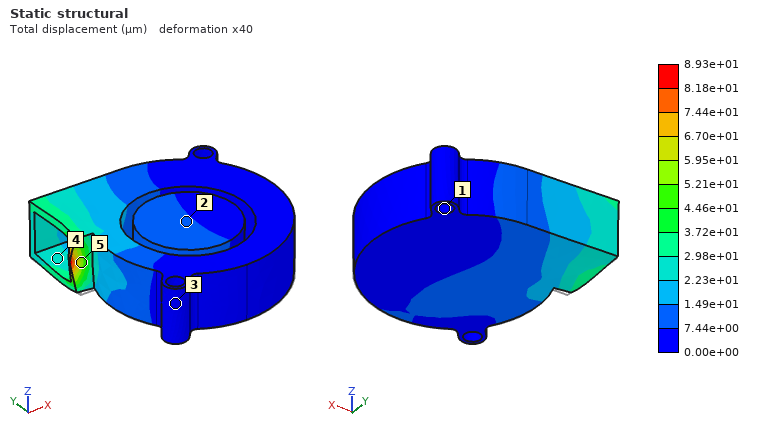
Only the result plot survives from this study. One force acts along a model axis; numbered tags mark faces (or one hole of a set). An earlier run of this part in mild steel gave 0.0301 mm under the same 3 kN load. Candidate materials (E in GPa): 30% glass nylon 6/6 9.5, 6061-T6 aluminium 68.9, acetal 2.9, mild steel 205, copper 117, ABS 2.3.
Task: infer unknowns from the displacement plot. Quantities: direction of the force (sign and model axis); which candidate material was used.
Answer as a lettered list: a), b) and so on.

a) +Y
b) 6061-T6 aluminium
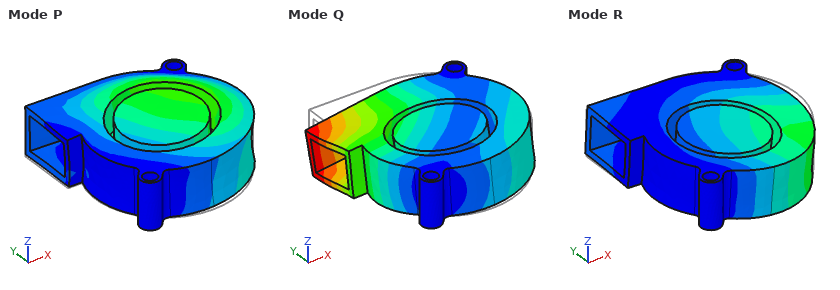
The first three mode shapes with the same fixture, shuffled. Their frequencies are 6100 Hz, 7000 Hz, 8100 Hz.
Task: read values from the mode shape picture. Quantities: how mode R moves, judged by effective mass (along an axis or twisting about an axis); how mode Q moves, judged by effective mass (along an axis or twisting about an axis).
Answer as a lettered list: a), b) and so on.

a) along Z
b) along Z
